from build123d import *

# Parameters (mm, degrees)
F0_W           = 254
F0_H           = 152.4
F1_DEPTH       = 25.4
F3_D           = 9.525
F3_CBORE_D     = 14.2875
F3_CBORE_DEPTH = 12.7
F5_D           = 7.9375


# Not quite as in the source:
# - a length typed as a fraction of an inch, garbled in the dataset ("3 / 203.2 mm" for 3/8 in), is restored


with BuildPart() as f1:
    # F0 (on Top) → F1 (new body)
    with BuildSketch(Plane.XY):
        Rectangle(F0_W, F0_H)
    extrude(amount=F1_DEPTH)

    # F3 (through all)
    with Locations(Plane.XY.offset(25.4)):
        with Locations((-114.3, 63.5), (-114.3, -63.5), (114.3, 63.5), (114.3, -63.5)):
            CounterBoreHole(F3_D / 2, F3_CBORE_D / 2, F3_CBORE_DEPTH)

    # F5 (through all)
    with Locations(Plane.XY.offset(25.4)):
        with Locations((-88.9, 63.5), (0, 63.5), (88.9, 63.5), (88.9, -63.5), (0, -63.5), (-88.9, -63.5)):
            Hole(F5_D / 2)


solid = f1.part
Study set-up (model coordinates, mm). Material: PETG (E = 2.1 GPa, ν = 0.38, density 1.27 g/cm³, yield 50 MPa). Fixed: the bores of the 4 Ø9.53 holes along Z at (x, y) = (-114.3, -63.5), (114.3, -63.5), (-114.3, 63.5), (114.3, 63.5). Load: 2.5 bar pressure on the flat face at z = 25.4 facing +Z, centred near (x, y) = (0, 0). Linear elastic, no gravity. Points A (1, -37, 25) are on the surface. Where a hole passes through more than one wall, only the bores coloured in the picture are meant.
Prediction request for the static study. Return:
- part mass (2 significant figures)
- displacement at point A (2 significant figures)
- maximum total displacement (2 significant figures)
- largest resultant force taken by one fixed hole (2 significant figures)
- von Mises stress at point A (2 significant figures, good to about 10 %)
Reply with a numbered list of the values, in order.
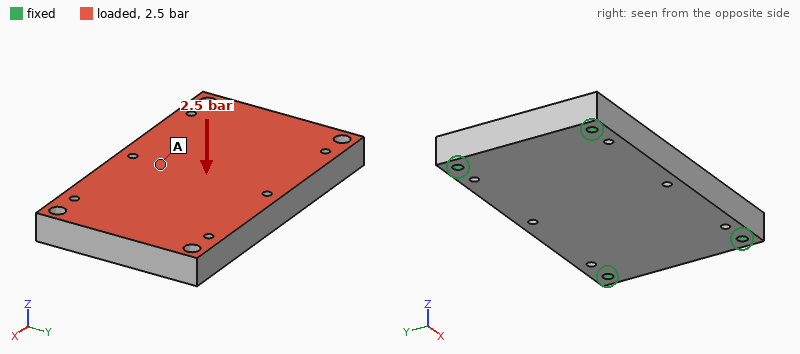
1. 1.2 kg
2. 1.6 mm
3. 1.7 mm
4. 3.2 kN
5. 9.0 MPa
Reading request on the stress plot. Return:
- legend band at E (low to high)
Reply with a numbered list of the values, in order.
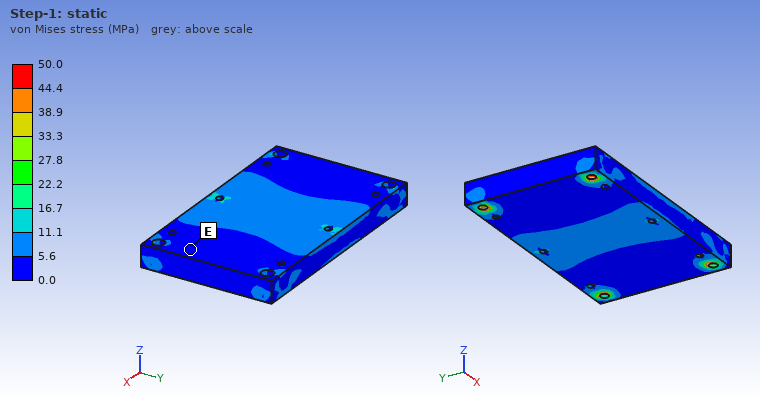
1. 0.0 to 5.6 MPa
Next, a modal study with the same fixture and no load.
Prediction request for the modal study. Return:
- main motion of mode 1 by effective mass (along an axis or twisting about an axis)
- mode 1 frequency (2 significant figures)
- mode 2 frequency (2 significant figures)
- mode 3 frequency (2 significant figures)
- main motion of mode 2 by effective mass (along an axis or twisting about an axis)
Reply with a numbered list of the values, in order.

1. along Z
2. 390 Hz
3. 680 Hz
4. 1000 Hz
5. twisting about X
